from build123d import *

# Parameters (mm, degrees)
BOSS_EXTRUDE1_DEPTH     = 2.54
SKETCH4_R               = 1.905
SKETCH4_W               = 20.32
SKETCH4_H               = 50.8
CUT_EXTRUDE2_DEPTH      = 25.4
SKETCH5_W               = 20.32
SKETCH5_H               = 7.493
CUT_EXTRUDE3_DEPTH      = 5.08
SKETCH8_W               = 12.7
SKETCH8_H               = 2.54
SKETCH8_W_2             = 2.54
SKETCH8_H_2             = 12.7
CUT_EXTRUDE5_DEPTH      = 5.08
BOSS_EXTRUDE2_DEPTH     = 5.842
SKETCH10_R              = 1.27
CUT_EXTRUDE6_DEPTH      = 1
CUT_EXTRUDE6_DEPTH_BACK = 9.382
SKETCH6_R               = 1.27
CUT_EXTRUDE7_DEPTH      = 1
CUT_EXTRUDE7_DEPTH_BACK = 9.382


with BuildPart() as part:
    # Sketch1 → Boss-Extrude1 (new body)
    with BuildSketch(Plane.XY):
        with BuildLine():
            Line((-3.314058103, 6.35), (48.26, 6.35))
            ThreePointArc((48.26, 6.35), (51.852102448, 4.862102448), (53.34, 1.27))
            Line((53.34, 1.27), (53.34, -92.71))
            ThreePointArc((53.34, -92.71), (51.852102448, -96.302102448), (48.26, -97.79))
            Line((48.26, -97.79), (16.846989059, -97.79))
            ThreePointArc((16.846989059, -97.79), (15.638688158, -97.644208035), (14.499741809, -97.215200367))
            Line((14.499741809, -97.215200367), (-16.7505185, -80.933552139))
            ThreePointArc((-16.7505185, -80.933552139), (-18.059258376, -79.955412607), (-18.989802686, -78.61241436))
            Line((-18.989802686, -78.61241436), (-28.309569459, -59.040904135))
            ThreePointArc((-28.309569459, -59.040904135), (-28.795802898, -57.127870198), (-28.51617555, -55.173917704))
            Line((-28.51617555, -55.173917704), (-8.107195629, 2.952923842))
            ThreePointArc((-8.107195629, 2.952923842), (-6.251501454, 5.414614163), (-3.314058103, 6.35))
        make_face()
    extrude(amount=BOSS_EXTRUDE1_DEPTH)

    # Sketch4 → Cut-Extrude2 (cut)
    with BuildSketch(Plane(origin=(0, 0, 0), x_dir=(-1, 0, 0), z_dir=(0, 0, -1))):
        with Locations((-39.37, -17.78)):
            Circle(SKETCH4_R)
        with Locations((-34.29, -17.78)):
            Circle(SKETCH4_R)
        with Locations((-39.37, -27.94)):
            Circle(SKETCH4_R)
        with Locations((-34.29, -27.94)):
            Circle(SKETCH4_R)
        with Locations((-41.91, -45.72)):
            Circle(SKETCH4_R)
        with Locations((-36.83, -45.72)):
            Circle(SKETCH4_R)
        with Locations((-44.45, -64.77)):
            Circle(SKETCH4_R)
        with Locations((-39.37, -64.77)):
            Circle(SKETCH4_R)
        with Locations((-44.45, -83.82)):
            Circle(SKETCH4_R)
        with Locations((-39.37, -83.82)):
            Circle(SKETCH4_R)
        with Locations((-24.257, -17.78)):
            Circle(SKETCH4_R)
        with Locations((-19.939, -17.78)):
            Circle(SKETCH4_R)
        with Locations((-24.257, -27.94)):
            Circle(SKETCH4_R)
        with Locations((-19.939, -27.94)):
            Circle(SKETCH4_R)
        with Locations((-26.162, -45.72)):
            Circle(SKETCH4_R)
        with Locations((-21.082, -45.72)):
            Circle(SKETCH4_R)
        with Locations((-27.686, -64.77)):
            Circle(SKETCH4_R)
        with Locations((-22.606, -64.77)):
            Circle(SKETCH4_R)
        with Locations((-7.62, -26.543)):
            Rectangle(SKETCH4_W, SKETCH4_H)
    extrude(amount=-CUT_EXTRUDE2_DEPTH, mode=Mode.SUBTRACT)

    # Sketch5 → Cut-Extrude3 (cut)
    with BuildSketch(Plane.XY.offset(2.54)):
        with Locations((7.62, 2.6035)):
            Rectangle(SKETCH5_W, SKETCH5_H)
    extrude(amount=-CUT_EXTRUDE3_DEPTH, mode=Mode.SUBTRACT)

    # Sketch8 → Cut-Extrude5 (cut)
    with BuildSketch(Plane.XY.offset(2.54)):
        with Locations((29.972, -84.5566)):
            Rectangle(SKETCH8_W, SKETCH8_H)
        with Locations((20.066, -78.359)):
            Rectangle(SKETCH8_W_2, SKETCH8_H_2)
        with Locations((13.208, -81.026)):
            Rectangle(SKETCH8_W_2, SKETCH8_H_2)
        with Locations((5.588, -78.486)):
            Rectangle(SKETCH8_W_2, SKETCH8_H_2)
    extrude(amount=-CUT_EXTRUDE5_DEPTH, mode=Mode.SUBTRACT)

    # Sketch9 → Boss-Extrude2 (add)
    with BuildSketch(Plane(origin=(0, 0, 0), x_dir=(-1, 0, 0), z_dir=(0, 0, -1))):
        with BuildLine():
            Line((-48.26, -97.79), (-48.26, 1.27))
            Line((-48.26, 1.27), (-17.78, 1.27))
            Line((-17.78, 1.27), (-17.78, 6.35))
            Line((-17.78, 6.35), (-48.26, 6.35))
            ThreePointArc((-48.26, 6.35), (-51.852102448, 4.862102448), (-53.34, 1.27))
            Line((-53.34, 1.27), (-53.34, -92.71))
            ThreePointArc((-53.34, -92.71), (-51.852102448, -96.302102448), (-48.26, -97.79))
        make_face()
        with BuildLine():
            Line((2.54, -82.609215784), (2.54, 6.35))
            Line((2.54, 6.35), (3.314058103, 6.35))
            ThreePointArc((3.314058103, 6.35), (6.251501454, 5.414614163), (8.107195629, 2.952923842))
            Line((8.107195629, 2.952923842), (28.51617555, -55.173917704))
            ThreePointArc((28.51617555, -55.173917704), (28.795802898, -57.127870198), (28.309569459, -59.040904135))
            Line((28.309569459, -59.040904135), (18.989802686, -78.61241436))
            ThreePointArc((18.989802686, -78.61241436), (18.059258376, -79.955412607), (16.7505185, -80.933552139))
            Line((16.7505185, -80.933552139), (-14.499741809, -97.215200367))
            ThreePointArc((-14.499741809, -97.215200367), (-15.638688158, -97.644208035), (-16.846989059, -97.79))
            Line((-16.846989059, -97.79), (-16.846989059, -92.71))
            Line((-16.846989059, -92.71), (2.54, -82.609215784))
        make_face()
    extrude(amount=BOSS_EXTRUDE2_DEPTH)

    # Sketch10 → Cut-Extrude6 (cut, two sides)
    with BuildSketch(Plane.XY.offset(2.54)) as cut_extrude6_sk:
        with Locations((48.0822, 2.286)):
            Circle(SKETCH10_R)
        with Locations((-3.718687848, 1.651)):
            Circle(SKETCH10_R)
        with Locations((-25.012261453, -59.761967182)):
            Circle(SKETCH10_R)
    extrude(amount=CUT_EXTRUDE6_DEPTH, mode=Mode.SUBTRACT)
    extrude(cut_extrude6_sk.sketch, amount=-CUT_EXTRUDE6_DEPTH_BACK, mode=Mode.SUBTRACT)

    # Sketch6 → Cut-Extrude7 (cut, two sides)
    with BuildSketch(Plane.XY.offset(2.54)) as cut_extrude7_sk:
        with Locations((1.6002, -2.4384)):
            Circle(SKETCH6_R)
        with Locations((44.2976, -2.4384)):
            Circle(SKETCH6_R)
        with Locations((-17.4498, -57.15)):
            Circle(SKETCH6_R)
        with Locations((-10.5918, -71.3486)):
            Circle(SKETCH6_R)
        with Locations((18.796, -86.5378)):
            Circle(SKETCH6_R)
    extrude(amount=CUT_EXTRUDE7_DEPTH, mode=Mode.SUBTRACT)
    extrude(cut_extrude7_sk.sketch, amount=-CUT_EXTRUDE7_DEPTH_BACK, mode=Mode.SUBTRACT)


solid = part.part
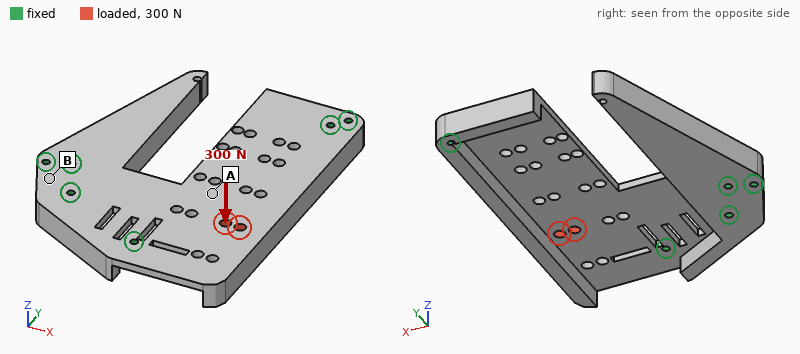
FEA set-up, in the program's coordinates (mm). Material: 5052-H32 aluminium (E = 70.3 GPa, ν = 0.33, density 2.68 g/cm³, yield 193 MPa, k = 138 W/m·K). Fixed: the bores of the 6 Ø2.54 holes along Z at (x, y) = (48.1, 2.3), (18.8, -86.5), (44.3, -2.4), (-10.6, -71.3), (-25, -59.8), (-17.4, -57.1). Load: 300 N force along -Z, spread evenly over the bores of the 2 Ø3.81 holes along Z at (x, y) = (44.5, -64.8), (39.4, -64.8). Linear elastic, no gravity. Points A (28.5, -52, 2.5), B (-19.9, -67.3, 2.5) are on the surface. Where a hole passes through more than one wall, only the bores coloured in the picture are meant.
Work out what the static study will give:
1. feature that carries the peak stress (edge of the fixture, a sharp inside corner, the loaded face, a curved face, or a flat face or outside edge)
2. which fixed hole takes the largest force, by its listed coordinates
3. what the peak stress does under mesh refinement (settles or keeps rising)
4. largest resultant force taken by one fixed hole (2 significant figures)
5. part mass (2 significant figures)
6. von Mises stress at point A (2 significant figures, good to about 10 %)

edge of the fixture
(48.1, 2.3)
keeps rising
660 N
75 g
23 MPa
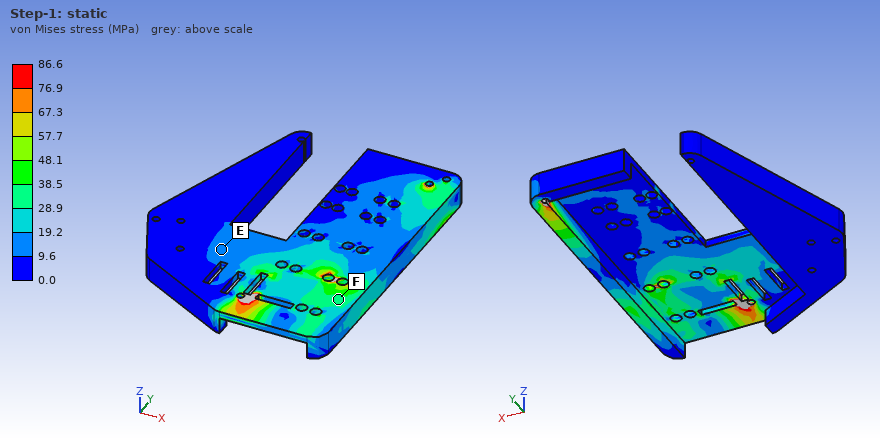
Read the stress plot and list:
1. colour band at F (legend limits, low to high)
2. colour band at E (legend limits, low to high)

28.9 to 38.5 MPa
9.6 to 19.2 MPa
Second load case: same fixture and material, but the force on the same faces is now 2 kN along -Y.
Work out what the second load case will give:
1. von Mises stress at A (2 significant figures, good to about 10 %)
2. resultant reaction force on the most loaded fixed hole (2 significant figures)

8.5 MPa
760 N
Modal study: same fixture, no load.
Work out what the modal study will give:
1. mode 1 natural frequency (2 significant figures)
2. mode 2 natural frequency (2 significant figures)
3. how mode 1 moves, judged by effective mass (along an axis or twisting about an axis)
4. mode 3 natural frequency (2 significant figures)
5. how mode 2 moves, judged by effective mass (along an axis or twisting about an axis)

1500 Hz
2500 Hz
along Z
3000 Hz
along Z
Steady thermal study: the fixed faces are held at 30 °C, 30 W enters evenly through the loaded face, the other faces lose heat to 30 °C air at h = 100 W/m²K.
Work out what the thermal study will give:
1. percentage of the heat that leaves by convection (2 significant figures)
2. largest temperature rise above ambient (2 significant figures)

52 %
55 K
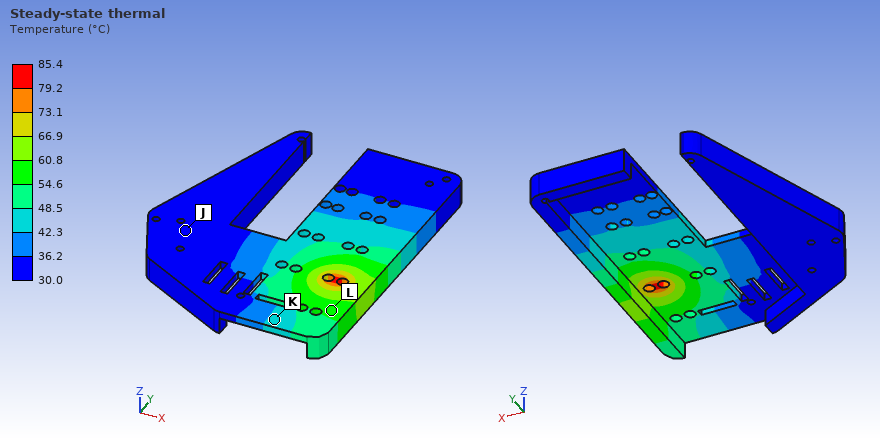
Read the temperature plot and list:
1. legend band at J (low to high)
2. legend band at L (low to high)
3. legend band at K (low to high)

30.0 to 36.2 °C
54.6 to 60.8 °C
42.3 to 48.5 °C
